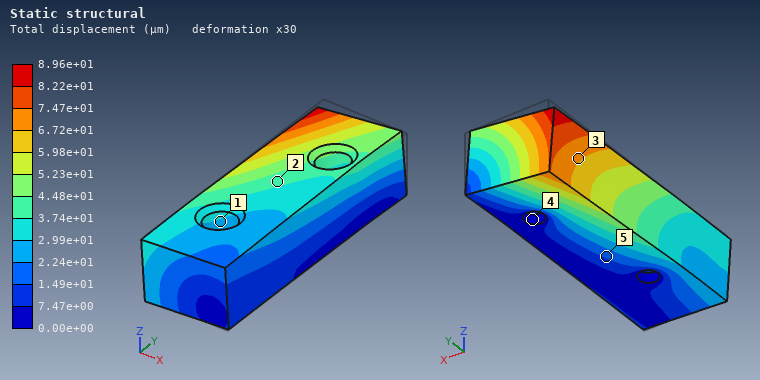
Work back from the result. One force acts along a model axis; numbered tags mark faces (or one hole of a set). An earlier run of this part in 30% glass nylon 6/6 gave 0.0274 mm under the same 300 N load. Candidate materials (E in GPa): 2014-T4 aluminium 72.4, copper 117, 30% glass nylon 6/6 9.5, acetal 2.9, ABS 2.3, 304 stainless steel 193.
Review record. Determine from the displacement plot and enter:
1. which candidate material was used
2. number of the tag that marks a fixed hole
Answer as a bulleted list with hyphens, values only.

- acetal
- 4
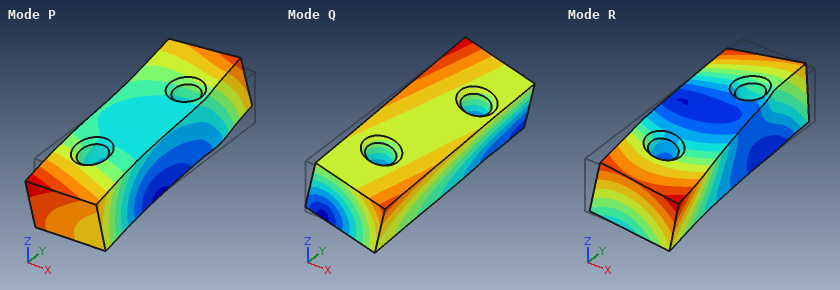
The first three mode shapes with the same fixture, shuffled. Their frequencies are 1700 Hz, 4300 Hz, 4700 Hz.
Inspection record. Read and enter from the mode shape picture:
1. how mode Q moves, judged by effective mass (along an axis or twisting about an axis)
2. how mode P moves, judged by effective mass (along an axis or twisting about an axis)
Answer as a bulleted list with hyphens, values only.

- along X
- along Y
